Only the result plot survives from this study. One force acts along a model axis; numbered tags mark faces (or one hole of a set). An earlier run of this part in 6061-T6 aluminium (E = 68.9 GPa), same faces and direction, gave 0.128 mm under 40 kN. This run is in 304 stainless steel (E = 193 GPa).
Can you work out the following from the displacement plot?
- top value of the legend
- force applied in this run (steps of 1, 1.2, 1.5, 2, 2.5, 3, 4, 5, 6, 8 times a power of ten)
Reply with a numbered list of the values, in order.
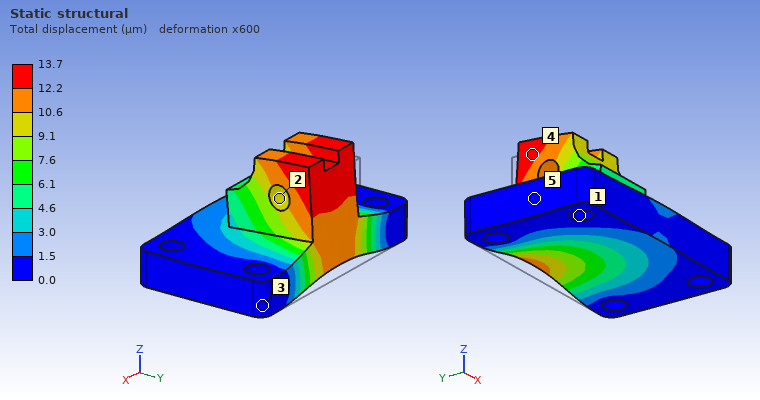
1. 13.7 µm
2. 12 kN
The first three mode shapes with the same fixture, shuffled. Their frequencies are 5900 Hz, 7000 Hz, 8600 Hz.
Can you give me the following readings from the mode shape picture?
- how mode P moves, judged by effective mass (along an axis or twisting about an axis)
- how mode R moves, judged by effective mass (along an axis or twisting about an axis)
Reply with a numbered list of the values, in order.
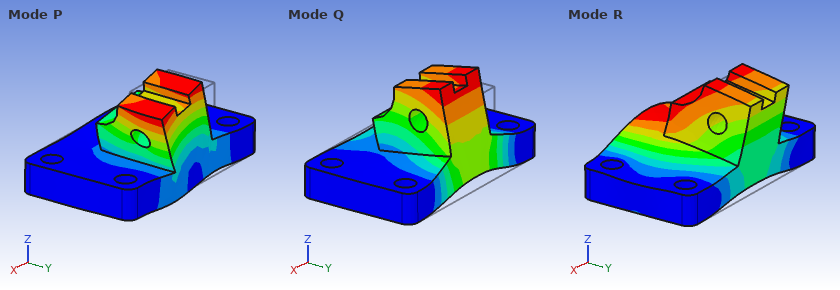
1. along X
2. along Z
